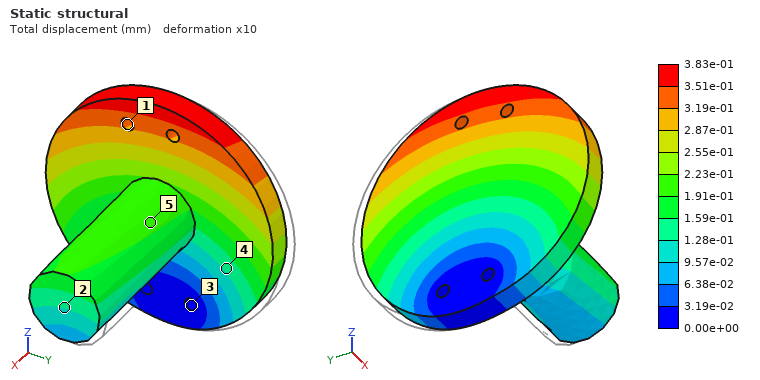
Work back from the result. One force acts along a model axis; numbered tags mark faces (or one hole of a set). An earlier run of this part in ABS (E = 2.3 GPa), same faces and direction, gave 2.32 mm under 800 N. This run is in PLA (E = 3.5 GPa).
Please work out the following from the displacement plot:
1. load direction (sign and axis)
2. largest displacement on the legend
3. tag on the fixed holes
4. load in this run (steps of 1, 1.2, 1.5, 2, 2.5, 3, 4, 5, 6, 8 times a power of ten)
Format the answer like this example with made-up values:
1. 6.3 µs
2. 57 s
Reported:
1. -Y
2. 3.83e-01 mm
3. 3
4. 200 N
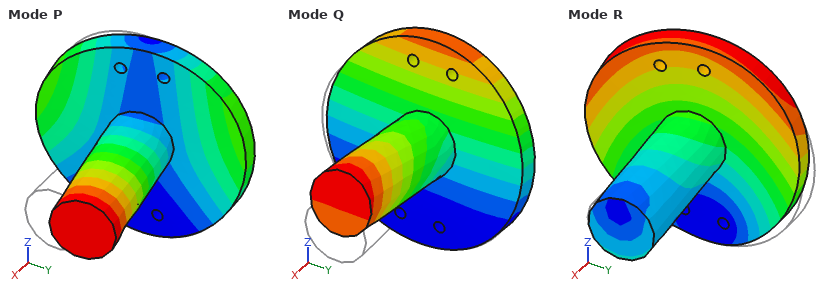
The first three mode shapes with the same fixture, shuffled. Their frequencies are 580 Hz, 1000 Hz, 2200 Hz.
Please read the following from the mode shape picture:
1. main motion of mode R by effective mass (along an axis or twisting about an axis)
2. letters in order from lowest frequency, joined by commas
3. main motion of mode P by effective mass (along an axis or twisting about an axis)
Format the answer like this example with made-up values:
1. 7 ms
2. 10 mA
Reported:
1. along Y
2. Q, P, R
3. along Y
